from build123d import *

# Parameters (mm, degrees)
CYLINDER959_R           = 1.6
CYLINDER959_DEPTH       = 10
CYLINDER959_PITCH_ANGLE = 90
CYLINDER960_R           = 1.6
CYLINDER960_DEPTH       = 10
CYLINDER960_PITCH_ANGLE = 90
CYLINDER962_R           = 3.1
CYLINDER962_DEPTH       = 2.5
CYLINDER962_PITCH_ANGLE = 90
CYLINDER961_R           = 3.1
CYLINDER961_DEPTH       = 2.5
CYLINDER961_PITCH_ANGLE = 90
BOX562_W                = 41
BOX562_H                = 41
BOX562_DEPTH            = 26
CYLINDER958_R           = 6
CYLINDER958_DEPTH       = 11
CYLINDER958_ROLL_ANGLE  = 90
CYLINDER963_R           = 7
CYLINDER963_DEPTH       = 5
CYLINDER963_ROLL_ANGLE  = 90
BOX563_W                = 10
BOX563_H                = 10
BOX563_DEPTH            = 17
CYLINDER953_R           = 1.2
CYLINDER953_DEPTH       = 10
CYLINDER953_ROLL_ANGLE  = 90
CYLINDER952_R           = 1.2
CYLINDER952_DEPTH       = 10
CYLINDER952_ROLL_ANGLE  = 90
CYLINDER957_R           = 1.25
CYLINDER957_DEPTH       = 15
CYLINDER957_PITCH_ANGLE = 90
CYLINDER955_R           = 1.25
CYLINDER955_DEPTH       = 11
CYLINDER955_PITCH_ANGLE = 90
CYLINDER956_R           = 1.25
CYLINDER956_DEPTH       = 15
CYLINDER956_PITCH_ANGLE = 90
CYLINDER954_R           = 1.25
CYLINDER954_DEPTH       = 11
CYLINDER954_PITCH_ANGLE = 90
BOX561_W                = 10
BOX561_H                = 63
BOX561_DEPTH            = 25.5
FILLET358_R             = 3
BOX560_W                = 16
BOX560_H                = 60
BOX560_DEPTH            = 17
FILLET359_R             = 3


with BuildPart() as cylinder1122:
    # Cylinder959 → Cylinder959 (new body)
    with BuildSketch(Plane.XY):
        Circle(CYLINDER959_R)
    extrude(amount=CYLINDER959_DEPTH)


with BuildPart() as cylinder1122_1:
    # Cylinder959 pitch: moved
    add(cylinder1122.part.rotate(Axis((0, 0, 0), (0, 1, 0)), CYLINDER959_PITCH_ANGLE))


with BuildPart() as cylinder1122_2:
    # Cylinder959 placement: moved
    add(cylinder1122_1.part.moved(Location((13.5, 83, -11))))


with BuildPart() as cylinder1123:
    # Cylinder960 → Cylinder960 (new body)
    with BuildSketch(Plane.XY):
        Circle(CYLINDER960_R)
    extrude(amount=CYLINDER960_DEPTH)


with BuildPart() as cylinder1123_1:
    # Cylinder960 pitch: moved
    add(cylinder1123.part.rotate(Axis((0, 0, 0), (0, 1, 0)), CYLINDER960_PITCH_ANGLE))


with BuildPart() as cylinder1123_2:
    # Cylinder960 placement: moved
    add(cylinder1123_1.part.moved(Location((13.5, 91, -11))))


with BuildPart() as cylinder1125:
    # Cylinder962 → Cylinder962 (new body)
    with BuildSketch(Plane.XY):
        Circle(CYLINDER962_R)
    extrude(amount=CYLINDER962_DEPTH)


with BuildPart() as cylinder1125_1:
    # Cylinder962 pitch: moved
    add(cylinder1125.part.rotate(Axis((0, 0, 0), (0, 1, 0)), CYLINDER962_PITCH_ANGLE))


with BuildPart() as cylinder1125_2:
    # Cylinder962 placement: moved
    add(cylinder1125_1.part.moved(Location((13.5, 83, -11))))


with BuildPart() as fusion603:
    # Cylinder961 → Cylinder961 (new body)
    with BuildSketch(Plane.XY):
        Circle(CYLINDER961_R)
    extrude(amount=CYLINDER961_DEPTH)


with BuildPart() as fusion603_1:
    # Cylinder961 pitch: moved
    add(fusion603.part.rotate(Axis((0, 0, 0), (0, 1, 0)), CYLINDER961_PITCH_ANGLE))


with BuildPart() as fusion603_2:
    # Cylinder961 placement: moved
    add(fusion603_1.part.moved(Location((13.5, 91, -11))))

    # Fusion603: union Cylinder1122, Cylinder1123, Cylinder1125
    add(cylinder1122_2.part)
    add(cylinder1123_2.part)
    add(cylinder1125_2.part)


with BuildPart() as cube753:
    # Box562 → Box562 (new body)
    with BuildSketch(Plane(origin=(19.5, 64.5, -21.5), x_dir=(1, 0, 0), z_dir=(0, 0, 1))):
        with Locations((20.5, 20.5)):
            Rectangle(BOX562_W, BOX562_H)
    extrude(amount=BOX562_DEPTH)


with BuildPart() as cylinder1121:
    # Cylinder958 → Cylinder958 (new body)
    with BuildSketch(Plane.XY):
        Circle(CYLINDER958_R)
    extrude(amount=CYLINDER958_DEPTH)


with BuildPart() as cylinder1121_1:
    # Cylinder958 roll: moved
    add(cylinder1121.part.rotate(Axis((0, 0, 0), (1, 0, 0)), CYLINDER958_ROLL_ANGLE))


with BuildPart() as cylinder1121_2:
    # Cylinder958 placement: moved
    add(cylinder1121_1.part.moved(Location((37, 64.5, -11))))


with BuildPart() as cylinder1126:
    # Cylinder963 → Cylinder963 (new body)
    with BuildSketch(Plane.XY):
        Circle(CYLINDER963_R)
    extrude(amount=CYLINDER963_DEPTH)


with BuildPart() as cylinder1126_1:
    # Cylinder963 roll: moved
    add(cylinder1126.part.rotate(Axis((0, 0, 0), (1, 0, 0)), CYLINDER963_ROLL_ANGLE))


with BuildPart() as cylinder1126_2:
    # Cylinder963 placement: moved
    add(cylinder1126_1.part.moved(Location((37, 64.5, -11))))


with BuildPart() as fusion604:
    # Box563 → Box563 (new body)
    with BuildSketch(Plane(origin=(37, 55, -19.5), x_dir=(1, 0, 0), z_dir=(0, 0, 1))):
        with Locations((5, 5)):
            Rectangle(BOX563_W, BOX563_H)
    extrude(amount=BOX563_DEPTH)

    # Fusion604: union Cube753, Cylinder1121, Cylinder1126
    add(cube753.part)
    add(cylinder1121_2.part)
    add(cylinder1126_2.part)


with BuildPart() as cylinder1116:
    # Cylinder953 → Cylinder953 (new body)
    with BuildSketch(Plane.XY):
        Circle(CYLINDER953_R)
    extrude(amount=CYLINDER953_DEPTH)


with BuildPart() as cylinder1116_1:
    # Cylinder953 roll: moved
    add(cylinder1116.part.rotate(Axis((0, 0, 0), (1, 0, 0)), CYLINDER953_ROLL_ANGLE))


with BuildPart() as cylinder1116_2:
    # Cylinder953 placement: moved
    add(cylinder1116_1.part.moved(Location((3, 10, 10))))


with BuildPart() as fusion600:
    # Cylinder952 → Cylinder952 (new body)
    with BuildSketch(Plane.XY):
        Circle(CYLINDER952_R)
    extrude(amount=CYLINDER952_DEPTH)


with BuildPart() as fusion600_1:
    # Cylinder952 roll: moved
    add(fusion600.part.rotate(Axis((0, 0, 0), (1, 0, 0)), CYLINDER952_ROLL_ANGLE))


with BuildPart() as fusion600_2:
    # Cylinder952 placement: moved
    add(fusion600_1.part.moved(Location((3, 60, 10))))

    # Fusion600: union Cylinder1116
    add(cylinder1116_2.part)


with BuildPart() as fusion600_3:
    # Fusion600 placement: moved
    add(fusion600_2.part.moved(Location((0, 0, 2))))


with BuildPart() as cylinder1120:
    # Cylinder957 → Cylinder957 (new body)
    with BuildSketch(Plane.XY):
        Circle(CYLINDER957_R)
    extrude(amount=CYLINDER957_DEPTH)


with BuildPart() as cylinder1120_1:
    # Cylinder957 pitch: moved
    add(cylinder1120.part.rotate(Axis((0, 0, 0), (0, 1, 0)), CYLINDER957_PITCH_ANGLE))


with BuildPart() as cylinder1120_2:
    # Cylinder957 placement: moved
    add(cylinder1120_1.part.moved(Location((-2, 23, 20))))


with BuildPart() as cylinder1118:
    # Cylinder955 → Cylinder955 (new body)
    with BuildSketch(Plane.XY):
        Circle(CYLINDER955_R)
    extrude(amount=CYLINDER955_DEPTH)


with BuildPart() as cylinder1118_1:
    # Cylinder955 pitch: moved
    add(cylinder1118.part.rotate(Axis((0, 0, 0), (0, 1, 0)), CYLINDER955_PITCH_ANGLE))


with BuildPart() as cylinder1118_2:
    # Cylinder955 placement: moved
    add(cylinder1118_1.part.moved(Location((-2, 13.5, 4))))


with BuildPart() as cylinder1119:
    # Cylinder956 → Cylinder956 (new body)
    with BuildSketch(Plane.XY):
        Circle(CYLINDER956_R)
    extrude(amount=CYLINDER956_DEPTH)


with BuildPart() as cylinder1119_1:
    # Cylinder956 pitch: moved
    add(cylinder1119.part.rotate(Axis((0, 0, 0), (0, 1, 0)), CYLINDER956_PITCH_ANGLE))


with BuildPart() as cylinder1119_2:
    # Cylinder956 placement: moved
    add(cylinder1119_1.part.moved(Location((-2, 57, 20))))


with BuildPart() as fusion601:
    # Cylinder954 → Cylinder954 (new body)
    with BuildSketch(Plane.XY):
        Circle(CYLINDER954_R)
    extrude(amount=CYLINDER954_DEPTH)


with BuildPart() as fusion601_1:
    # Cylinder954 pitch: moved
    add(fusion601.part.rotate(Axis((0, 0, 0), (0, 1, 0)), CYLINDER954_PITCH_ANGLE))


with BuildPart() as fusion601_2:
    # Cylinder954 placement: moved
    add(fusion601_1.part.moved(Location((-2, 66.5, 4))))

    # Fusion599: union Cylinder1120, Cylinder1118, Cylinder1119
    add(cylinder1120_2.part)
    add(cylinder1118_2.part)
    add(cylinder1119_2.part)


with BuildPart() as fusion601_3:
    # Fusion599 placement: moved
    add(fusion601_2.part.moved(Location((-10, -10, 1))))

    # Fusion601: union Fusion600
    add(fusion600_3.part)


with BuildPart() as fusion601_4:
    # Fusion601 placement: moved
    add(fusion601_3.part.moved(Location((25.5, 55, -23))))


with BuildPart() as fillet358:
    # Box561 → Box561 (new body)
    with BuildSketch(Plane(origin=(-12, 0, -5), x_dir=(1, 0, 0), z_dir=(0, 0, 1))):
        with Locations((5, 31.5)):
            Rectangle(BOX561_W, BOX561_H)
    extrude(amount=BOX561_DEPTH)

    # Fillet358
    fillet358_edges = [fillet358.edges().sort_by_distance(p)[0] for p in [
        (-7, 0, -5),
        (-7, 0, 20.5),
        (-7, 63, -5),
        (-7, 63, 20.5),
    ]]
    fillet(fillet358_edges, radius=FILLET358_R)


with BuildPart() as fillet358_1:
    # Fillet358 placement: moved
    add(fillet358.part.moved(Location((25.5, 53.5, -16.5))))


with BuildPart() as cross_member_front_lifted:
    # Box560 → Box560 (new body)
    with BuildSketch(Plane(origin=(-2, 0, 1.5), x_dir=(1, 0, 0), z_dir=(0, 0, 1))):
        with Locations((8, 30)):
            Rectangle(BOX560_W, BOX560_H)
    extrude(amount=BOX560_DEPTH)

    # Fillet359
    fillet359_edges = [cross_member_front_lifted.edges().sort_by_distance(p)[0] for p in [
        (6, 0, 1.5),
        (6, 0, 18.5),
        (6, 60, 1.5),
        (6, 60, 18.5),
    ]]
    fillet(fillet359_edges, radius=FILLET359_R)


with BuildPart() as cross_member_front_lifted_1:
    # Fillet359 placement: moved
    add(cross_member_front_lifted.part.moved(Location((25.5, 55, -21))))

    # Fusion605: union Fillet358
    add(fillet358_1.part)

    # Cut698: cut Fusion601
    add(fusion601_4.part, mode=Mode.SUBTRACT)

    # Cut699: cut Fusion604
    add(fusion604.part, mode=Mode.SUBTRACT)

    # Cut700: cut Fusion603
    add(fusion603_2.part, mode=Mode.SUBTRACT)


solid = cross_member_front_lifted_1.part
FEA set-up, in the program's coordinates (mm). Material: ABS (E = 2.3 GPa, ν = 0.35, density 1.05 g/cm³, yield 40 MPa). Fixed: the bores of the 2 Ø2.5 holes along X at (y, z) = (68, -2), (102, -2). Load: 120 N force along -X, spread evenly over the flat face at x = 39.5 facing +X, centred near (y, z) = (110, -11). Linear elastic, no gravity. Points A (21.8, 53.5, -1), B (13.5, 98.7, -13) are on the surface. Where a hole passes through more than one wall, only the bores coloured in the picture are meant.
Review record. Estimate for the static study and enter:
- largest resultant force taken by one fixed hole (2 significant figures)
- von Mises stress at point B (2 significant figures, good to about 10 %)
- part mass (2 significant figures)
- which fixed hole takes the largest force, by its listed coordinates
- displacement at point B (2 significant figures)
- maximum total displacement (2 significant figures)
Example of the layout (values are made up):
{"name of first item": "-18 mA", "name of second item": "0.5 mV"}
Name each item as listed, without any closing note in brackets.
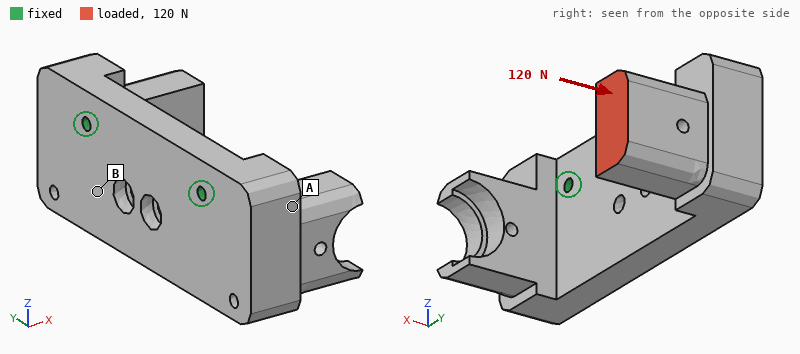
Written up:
{"largest resultant force taken by one fixed hole": "130 N", "von Mises stress at point B": "2.8 MPa", "part mass": "16 g", "which fixed hole takes the largest force, by its listed coordinates": "(102, -2)", "displacement at point B": "0.066 mm", "maximum total displacement": "0.34 mm"}
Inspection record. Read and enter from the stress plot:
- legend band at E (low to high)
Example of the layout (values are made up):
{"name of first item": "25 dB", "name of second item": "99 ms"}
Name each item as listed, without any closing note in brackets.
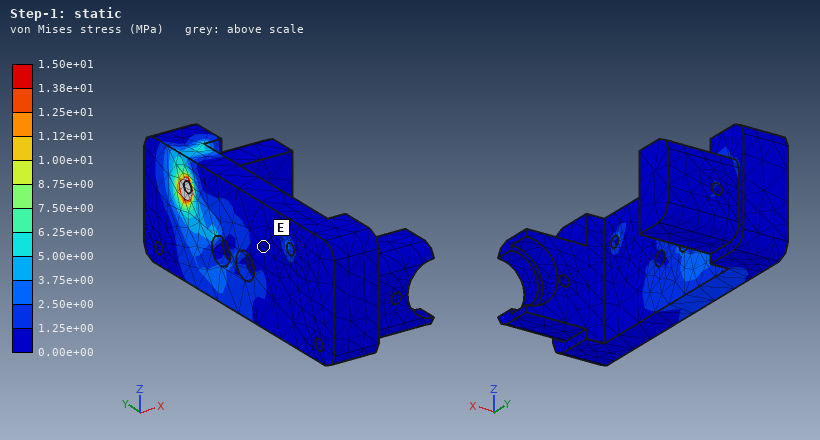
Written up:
{"legend band at E": "0.00e+00 to 1.25e+00 MPa"}
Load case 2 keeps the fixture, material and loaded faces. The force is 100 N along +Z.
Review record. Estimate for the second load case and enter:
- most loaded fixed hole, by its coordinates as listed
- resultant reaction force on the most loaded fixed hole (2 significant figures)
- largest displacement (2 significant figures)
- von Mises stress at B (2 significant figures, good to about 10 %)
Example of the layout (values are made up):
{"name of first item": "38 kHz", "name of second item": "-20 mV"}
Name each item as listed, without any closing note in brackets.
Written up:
{"most loaded fixed hole, by its coordinates as listed": "(102, -2)", "resultant reaction force on the most loaded fixed hole": "120 N", "largest displacement": "0.57 mm", "von Mises stress at B": "4.6 MPa"}
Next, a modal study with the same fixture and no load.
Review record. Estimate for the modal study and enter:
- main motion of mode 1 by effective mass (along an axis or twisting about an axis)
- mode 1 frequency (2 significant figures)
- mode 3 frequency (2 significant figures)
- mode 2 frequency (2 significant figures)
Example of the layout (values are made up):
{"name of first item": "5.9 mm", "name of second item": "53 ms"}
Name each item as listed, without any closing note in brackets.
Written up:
{"main motion of mode 1 by effective mass": "along X", "mode 1 frequency": "1400 Hz", "mode 3 frequency": "1900 Hz", "mode 2 frequency": "1700 Hz"}
